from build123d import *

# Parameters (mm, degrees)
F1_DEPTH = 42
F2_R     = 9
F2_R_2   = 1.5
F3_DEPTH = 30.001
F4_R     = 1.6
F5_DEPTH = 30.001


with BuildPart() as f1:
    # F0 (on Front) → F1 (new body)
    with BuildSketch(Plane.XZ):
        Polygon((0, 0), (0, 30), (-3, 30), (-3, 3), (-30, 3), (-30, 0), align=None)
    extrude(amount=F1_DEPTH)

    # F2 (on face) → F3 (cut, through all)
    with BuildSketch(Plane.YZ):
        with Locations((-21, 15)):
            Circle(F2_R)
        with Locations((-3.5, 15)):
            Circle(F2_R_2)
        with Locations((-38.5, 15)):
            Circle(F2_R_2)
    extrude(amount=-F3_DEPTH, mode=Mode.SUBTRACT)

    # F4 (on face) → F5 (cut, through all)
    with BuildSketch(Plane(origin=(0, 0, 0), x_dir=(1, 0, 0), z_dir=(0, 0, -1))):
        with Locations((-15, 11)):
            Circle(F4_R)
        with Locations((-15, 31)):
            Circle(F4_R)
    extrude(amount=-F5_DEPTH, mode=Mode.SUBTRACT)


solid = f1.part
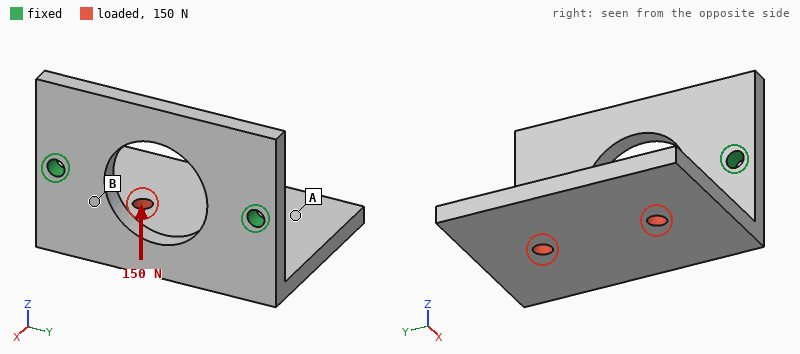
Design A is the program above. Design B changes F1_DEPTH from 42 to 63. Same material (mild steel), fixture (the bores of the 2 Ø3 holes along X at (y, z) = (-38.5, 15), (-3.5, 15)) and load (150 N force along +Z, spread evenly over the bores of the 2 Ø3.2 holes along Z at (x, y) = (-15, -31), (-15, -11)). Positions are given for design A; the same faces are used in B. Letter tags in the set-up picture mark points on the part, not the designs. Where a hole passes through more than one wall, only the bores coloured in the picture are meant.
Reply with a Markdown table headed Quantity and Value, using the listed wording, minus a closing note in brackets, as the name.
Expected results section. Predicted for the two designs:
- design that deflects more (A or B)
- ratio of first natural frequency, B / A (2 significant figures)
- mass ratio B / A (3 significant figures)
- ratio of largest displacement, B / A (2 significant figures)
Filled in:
| Quantity | Value |
|---|---|
| design that deflects more | A |
| ratio of first natural frequency, B / A | 0.97 |
| mass ratio B / A | 1.57 |
| ratio of largest displacement, B / A | 0.77 |
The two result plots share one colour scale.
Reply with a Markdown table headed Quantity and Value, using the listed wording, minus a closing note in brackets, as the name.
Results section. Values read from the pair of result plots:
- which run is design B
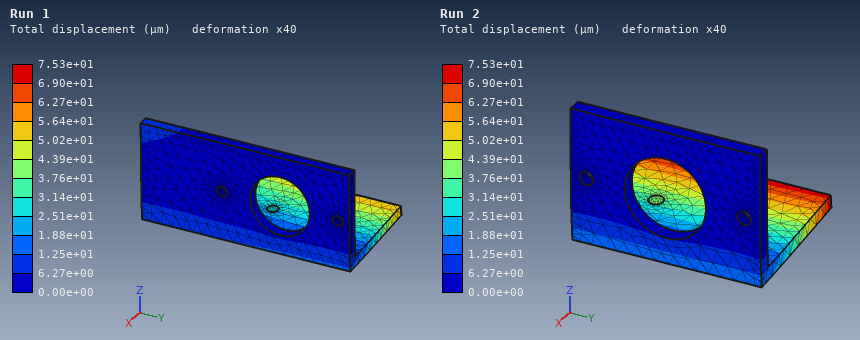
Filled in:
| Quantity | Value |
|---|---|
| which run is design B | Run 1 |
